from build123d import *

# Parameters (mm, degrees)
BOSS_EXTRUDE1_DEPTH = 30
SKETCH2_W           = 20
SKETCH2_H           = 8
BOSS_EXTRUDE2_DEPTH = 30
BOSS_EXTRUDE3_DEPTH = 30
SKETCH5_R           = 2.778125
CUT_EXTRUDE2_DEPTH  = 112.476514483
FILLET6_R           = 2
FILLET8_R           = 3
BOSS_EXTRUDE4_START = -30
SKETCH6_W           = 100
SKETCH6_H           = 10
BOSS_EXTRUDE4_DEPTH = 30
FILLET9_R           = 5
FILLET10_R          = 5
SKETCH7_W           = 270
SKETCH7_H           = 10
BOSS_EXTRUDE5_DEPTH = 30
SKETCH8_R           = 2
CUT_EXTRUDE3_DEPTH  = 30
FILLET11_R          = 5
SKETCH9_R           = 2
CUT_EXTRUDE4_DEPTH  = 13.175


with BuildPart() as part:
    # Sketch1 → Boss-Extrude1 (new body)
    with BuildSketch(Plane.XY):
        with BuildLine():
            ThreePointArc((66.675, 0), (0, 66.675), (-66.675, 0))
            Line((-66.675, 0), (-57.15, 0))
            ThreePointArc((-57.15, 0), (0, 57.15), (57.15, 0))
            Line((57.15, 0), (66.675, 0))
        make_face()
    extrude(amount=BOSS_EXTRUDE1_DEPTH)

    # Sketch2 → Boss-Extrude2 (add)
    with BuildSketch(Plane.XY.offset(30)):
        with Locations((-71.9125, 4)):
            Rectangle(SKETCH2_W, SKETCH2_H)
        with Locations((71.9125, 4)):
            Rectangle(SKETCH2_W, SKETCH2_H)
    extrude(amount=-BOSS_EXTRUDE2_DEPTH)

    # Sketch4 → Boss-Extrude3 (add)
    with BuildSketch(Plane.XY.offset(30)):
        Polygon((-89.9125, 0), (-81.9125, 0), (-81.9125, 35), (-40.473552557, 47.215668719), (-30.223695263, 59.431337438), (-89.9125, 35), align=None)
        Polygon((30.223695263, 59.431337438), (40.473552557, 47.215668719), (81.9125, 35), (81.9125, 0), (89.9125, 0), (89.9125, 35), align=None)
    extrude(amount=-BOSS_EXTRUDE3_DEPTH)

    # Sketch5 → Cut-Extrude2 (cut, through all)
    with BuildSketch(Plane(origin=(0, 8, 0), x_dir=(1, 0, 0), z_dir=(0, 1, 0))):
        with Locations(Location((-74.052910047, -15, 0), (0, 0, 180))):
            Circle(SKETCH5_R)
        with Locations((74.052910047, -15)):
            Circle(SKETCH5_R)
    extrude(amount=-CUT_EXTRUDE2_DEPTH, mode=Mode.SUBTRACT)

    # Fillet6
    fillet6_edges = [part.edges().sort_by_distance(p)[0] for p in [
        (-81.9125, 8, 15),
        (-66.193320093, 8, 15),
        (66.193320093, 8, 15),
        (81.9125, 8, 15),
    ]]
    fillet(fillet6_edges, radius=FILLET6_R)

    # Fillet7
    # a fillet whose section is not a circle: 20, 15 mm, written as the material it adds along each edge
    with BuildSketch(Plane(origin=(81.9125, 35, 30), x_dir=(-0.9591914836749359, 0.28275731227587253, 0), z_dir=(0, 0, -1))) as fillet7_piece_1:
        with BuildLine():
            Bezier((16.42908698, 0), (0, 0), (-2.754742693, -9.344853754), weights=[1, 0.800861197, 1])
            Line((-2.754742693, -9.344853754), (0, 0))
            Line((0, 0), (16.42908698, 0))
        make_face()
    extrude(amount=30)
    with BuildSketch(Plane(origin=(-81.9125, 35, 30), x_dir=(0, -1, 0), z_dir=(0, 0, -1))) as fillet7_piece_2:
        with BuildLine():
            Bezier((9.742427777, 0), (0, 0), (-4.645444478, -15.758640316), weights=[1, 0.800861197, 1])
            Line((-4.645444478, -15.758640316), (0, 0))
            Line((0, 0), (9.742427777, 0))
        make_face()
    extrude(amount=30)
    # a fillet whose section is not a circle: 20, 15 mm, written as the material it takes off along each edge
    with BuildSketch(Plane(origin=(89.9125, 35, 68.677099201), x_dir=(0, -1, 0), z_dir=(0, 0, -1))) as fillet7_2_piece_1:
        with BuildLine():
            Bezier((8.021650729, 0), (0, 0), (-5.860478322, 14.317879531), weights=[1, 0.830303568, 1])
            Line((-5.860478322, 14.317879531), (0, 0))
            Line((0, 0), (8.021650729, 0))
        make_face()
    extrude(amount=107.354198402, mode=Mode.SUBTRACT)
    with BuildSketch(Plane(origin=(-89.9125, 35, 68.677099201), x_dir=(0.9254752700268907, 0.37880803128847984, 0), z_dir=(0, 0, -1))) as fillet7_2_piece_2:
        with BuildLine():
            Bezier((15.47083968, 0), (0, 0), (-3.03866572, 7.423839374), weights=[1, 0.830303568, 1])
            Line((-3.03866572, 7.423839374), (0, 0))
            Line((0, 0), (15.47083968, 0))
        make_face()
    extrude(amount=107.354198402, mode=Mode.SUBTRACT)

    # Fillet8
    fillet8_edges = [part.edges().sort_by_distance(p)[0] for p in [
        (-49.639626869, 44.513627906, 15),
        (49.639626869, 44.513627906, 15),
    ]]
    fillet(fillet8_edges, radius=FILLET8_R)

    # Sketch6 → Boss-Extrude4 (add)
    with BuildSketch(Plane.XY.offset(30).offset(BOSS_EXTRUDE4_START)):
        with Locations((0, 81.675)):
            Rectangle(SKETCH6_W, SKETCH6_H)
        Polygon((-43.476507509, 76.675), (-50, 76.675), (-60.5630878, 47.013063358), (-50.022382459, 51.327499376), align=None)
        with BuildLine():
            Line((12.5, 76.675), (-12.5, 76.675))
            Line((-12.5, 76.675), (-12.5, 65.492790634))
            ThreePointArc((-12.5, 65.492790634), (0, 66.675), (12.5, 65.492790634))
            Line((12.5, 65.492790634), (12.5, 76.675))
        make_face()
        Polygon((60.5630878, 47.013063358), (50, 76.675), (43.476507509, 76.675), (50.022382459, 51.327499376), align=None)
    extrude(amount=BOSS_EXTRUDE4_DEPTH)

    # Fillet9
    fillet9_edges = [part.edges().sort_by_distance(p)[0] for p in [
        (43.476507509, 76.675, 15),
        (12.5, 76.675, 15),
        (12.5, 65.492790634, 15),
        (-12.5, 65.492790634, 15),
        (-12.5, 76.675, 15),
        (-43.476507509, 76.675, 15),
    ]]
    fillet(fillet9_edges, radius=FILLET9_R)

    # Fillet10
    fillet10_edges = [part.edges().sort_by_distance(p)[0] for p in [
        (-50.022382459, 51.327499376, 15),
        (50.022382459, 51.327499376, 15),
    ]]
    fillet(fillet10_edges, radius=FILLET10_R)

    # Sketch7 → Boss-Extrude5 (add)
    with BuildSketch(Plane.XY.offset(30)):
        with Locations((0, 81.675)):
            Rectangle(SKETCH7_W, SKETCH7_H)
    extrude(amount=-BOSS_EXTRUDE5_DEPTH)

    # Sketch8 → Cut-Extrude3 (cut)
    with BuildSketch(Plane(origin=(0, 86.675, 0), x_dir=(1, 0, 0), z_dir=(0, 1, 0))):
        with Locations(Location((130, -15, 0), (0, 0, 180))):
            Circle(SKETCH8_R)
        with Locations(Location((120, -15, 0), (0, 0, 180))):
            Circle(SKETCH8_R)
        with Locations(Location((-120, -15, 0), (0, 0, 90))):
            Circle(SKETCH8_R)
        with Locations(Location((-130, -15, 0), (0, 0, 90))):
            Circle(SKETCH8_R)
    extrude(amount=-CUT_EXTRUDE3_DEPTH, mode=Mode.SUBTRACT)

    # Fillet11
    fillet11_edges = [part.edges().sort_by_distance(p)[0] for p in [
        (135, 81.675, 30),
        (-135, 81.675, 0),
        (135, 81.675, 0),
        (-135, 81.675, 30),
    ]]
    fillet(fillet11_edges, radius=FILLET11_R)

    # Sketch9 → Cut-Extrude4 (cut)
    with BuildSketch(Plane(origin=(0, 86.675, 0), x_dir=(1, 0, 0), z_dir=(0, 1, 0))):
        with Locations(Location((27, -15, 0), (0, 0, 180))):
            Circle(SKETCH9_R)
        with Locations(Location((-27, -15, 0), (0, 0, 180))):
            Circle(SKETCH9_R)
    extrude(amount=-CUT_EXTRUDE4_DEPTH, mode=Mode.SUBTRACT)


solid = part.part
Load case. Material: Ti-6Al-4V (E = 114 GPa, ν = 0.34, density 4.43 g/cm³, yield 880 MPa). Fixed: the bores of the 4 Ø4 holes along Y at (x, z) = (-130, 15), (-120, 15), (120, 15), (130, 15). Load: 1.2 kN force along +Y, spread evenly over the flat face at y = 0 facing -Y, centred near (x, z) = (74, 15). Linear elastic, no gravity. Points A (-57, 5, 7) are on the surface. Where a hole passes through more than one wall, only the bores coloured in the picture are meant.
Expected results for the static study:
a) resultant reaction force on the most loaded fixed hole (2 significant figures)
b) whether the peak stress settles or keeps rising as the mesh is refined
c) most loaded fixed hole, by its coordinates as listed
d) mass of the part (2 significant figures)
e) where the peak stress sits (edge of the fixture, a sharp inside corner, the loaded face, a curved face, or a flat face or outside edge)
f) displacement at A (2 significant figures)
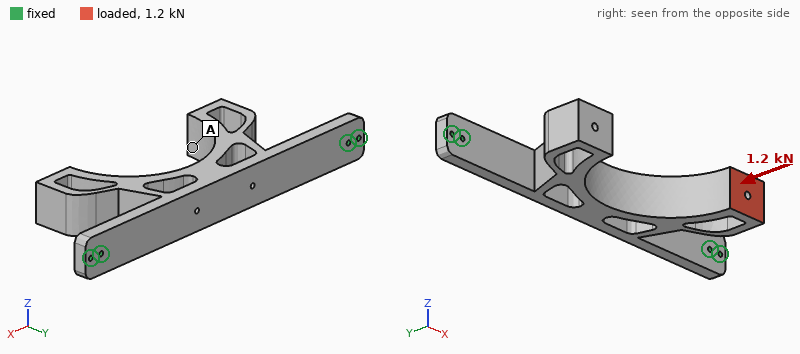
2.2 kN
keeps rising
(120, 15)
870 g
edge of the fixture
0.091 mm
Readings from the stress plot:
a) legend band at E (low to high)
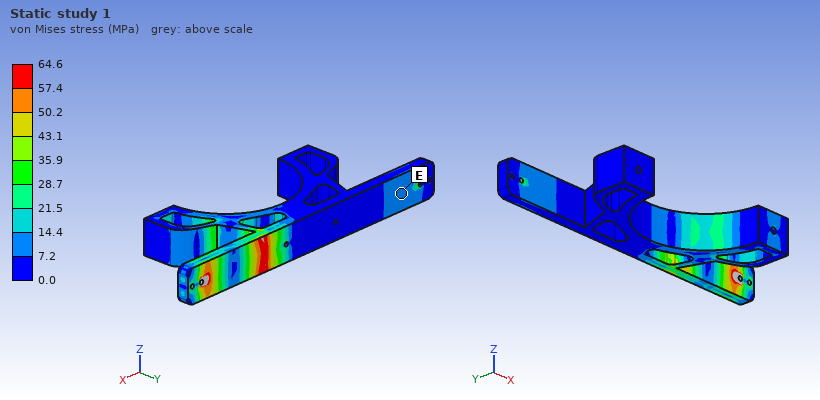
7.2 to 14.4 MPa
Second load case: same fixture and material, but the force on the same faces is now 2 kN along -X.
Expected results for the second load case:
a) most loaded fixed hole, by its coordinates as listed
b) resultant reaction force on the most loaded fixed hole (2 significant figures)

(-120, 15)
2.2 kN
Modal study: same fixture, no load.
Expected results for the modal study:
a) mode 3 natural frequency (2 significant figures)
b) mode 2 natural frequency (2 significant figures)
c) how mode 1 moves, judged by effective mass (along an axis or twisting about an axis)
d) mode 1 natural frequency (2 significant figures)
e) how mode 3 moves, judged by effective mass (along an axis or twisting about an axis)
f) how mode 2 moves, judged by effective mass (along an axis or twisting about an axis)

810 Hz
640 Hz
along Z
420 Hz
along X
along Y
